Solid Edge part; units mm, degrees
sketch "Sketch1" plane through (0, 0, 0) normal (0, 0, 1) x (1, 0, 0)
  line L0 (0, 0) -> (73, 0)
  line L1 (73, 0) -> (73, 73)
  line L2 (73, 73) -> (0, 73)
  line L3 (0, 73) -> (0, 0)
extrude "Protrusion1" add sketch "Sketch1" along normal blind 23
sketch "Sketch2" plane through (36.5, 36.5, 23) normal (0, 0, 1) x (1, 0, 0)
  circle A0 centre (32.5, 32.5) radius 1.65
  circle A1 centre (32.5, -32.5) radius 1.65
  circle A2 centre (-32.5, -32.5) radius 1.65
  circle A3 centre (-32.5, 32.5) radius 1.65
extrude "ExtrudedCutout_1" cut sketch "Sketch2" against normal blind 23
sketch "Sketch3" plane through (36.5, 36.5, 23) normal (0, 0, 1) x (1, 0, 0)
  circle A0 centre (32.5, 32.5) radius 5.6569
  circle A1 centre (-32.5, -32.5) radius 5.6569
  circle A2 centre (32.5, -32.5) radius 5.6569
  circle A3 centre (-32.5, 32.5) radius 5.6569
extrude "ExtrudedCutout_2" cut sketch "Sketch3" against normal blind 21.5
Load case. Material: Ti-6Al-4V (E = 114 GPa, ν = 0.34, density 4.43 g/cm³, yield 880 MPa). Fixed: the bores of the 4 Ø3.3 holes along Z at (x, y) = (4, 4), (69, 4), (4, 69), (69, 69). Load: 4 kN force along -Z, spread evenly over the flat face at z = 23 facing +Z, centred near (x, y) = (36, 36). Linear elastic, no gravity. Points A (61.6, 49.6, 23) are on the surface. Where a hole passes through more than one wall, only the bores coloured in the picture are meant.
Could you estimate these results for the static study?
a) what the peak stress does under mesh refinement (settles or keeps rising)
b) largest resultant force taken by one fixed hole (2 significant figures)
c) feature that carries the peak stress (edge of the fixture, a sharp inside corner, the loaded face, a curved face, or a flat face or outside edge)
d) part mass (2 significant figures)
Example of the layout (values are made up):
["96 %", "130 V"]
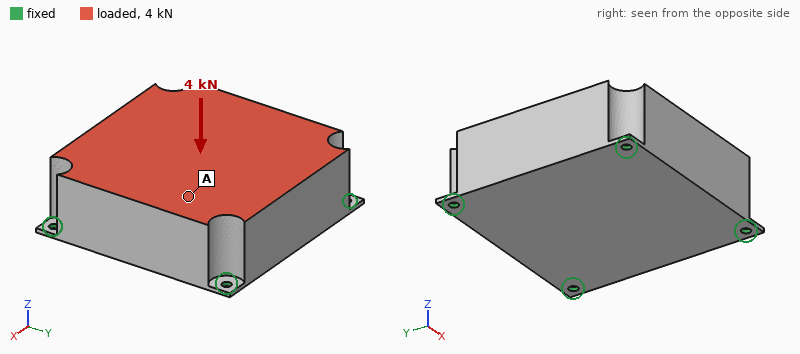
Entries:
["keeps rising", "1.1 kN", "edge of the fixture", "510 g"]
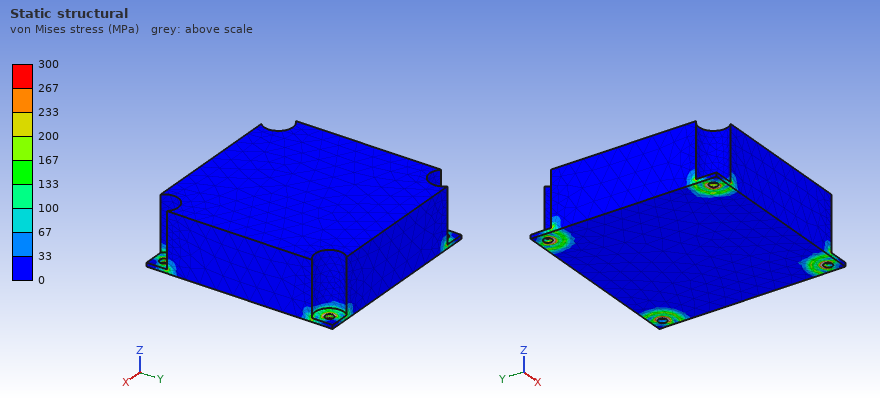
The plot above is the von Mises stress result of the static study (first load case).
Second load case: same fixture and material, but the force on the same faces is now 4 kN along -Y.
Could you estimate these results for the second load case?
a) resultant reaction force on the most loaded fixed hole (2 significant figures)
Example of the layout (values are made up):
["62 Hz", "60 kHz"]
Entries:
["1.3 kN"]
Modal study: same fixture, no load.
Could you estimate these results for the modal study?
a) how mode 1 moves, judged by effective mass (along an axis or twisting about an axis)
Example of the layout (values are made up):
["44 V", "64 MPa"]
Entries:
["along Z"]
